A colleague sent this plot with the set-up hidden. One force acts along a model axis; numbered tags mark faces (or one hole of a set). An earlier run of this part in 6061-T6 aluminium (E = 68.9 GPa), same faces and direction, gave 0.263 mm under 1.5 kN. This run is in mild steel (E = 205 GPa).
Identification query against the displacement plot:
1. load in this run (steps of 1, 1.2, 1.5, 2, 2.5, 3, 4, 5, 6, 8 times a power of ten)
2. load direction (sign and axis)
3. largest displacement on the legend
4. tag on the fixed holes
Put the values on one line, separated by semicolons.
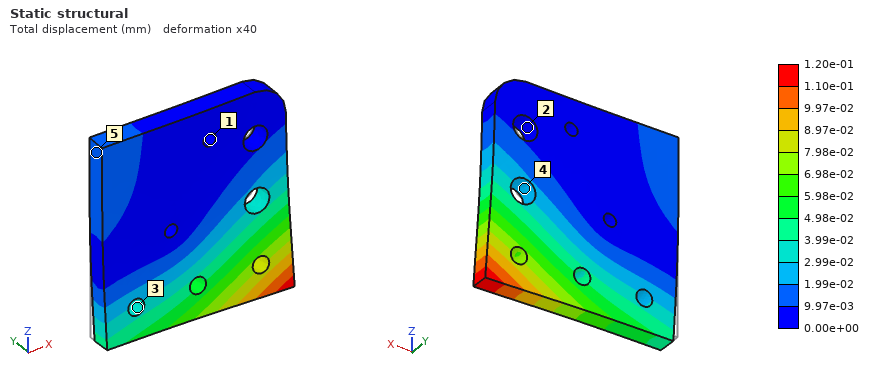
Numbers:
2 kN; -Y; 1.20e-01 mm; 1
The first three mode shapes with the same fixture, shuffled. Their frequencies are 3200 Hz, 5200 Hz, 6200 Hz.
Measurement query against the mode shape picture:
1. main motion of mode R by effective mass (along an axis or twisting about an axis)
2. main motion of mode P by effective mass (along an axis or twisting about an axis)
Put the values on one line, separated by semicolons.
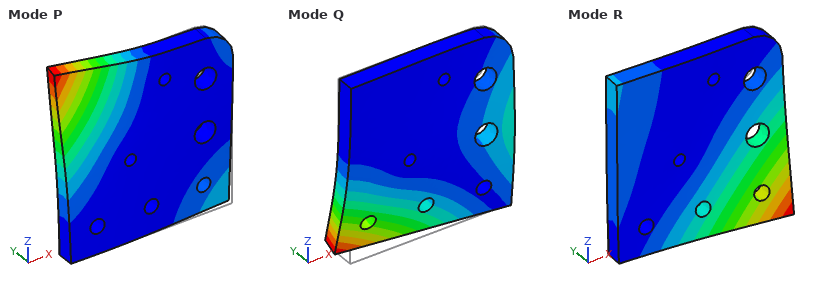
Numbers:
along Y; along Y
